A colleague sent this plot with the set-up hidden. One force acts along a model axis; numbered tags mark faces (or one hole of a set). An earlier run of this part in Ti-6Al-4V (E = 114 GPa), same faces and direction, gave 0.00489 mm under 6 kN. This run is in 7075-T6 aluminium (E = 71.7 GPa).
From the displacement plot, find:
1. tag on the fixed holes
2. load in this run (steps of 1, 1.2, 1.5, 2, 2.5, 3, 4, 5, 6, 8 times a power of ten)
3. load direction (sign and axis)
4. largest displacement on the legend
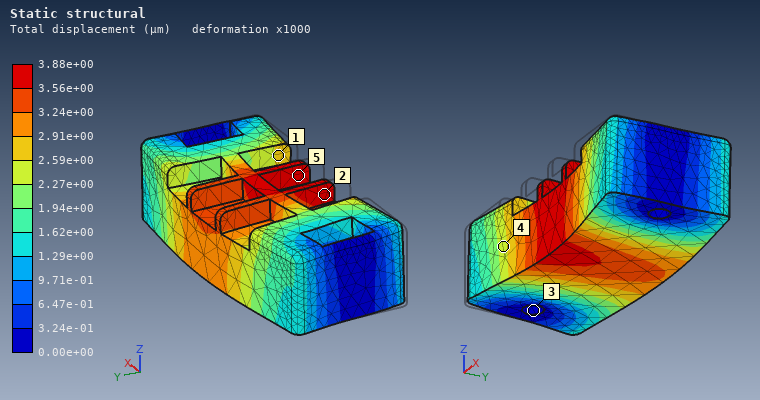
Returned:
3
3 kN
+Y
3.88e+00 µm
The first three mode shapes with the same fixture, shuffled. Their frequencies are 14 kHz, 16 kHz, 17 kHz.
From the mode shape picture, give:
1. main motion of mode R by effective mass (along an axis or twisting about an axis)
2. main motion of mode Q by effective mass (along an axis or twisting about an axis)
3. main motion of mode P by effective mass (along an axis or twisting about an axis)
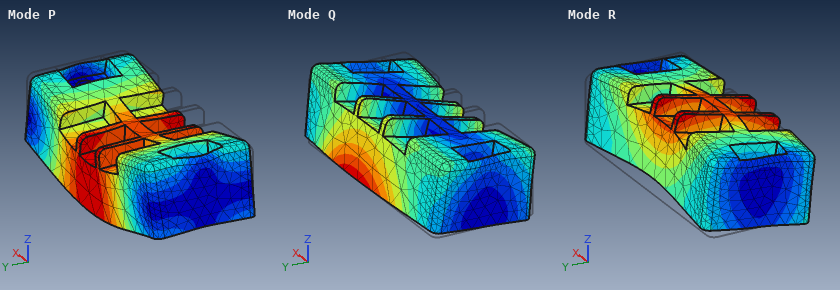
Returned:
along Y
along Y
along Z
